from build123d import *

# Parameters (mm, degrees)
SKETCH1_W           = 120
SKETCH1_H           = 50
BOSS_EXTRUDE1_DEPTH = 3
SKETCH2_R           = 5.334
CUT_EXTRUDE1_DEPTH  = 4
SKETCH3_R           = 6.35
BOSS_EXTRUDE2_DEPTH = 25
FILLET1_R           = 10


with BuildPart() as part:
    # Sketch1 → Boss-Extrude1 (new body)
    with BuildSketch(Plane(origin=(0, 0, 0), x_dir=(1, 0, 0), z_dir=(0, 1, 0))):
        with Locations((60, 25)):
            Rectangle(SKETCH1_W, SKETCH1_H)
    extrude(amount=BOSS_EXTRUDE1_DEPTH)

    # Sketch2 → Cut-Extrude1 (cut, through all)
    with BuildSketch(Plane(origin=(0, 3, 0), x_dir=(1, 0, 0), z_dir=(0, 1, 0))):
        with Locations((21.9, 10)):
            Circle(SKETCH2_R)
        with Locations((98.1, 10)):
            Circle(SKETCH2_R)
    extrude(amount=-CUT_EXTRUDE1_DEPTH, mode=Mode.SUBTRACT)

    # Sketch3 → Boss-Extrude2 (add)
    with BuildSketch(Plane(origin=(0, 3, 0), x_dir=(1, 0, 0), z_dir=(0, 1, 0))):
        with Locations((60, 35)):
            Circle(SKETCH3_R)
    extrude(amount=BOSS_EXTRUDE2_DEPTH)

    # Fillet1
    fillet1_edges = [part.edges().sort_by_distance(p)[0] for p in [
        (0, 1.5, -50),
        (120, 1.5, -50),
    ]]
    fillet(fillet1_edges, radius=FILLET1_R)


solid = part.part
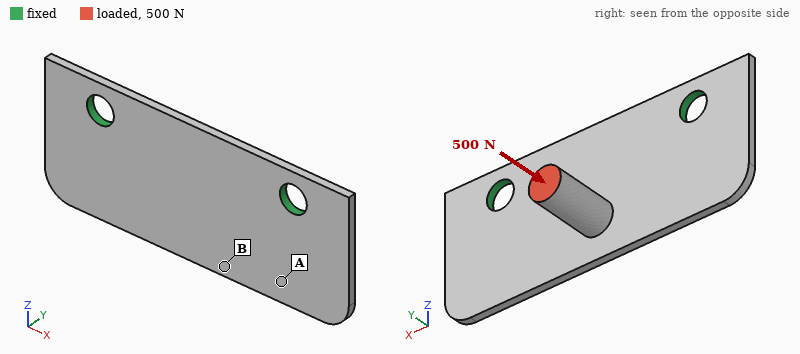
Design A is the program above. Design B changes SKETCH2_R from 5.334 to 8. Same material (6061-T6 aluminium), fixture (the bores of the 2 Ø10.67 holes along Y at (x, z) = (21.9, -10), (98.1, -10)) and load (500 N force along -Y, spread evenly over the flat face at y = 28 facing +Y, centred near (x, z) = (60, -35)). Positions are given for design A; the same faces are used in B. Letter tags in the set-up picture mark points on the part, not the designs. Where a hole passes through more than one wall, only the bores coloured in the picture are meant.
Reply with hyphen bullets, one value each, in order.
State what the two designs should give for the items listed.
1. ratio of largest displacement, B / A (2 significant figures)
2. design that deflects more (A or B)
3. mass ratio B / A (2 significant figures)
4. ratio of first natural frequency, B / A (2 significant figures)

- 0.79
- A
- 0.97
- 1.2
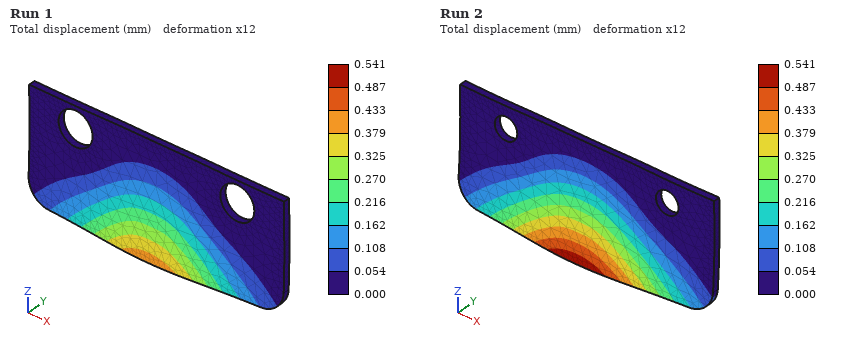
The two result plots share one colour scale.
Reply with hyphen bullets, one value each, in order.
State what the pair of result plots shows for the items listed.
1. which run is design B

- Run 1
